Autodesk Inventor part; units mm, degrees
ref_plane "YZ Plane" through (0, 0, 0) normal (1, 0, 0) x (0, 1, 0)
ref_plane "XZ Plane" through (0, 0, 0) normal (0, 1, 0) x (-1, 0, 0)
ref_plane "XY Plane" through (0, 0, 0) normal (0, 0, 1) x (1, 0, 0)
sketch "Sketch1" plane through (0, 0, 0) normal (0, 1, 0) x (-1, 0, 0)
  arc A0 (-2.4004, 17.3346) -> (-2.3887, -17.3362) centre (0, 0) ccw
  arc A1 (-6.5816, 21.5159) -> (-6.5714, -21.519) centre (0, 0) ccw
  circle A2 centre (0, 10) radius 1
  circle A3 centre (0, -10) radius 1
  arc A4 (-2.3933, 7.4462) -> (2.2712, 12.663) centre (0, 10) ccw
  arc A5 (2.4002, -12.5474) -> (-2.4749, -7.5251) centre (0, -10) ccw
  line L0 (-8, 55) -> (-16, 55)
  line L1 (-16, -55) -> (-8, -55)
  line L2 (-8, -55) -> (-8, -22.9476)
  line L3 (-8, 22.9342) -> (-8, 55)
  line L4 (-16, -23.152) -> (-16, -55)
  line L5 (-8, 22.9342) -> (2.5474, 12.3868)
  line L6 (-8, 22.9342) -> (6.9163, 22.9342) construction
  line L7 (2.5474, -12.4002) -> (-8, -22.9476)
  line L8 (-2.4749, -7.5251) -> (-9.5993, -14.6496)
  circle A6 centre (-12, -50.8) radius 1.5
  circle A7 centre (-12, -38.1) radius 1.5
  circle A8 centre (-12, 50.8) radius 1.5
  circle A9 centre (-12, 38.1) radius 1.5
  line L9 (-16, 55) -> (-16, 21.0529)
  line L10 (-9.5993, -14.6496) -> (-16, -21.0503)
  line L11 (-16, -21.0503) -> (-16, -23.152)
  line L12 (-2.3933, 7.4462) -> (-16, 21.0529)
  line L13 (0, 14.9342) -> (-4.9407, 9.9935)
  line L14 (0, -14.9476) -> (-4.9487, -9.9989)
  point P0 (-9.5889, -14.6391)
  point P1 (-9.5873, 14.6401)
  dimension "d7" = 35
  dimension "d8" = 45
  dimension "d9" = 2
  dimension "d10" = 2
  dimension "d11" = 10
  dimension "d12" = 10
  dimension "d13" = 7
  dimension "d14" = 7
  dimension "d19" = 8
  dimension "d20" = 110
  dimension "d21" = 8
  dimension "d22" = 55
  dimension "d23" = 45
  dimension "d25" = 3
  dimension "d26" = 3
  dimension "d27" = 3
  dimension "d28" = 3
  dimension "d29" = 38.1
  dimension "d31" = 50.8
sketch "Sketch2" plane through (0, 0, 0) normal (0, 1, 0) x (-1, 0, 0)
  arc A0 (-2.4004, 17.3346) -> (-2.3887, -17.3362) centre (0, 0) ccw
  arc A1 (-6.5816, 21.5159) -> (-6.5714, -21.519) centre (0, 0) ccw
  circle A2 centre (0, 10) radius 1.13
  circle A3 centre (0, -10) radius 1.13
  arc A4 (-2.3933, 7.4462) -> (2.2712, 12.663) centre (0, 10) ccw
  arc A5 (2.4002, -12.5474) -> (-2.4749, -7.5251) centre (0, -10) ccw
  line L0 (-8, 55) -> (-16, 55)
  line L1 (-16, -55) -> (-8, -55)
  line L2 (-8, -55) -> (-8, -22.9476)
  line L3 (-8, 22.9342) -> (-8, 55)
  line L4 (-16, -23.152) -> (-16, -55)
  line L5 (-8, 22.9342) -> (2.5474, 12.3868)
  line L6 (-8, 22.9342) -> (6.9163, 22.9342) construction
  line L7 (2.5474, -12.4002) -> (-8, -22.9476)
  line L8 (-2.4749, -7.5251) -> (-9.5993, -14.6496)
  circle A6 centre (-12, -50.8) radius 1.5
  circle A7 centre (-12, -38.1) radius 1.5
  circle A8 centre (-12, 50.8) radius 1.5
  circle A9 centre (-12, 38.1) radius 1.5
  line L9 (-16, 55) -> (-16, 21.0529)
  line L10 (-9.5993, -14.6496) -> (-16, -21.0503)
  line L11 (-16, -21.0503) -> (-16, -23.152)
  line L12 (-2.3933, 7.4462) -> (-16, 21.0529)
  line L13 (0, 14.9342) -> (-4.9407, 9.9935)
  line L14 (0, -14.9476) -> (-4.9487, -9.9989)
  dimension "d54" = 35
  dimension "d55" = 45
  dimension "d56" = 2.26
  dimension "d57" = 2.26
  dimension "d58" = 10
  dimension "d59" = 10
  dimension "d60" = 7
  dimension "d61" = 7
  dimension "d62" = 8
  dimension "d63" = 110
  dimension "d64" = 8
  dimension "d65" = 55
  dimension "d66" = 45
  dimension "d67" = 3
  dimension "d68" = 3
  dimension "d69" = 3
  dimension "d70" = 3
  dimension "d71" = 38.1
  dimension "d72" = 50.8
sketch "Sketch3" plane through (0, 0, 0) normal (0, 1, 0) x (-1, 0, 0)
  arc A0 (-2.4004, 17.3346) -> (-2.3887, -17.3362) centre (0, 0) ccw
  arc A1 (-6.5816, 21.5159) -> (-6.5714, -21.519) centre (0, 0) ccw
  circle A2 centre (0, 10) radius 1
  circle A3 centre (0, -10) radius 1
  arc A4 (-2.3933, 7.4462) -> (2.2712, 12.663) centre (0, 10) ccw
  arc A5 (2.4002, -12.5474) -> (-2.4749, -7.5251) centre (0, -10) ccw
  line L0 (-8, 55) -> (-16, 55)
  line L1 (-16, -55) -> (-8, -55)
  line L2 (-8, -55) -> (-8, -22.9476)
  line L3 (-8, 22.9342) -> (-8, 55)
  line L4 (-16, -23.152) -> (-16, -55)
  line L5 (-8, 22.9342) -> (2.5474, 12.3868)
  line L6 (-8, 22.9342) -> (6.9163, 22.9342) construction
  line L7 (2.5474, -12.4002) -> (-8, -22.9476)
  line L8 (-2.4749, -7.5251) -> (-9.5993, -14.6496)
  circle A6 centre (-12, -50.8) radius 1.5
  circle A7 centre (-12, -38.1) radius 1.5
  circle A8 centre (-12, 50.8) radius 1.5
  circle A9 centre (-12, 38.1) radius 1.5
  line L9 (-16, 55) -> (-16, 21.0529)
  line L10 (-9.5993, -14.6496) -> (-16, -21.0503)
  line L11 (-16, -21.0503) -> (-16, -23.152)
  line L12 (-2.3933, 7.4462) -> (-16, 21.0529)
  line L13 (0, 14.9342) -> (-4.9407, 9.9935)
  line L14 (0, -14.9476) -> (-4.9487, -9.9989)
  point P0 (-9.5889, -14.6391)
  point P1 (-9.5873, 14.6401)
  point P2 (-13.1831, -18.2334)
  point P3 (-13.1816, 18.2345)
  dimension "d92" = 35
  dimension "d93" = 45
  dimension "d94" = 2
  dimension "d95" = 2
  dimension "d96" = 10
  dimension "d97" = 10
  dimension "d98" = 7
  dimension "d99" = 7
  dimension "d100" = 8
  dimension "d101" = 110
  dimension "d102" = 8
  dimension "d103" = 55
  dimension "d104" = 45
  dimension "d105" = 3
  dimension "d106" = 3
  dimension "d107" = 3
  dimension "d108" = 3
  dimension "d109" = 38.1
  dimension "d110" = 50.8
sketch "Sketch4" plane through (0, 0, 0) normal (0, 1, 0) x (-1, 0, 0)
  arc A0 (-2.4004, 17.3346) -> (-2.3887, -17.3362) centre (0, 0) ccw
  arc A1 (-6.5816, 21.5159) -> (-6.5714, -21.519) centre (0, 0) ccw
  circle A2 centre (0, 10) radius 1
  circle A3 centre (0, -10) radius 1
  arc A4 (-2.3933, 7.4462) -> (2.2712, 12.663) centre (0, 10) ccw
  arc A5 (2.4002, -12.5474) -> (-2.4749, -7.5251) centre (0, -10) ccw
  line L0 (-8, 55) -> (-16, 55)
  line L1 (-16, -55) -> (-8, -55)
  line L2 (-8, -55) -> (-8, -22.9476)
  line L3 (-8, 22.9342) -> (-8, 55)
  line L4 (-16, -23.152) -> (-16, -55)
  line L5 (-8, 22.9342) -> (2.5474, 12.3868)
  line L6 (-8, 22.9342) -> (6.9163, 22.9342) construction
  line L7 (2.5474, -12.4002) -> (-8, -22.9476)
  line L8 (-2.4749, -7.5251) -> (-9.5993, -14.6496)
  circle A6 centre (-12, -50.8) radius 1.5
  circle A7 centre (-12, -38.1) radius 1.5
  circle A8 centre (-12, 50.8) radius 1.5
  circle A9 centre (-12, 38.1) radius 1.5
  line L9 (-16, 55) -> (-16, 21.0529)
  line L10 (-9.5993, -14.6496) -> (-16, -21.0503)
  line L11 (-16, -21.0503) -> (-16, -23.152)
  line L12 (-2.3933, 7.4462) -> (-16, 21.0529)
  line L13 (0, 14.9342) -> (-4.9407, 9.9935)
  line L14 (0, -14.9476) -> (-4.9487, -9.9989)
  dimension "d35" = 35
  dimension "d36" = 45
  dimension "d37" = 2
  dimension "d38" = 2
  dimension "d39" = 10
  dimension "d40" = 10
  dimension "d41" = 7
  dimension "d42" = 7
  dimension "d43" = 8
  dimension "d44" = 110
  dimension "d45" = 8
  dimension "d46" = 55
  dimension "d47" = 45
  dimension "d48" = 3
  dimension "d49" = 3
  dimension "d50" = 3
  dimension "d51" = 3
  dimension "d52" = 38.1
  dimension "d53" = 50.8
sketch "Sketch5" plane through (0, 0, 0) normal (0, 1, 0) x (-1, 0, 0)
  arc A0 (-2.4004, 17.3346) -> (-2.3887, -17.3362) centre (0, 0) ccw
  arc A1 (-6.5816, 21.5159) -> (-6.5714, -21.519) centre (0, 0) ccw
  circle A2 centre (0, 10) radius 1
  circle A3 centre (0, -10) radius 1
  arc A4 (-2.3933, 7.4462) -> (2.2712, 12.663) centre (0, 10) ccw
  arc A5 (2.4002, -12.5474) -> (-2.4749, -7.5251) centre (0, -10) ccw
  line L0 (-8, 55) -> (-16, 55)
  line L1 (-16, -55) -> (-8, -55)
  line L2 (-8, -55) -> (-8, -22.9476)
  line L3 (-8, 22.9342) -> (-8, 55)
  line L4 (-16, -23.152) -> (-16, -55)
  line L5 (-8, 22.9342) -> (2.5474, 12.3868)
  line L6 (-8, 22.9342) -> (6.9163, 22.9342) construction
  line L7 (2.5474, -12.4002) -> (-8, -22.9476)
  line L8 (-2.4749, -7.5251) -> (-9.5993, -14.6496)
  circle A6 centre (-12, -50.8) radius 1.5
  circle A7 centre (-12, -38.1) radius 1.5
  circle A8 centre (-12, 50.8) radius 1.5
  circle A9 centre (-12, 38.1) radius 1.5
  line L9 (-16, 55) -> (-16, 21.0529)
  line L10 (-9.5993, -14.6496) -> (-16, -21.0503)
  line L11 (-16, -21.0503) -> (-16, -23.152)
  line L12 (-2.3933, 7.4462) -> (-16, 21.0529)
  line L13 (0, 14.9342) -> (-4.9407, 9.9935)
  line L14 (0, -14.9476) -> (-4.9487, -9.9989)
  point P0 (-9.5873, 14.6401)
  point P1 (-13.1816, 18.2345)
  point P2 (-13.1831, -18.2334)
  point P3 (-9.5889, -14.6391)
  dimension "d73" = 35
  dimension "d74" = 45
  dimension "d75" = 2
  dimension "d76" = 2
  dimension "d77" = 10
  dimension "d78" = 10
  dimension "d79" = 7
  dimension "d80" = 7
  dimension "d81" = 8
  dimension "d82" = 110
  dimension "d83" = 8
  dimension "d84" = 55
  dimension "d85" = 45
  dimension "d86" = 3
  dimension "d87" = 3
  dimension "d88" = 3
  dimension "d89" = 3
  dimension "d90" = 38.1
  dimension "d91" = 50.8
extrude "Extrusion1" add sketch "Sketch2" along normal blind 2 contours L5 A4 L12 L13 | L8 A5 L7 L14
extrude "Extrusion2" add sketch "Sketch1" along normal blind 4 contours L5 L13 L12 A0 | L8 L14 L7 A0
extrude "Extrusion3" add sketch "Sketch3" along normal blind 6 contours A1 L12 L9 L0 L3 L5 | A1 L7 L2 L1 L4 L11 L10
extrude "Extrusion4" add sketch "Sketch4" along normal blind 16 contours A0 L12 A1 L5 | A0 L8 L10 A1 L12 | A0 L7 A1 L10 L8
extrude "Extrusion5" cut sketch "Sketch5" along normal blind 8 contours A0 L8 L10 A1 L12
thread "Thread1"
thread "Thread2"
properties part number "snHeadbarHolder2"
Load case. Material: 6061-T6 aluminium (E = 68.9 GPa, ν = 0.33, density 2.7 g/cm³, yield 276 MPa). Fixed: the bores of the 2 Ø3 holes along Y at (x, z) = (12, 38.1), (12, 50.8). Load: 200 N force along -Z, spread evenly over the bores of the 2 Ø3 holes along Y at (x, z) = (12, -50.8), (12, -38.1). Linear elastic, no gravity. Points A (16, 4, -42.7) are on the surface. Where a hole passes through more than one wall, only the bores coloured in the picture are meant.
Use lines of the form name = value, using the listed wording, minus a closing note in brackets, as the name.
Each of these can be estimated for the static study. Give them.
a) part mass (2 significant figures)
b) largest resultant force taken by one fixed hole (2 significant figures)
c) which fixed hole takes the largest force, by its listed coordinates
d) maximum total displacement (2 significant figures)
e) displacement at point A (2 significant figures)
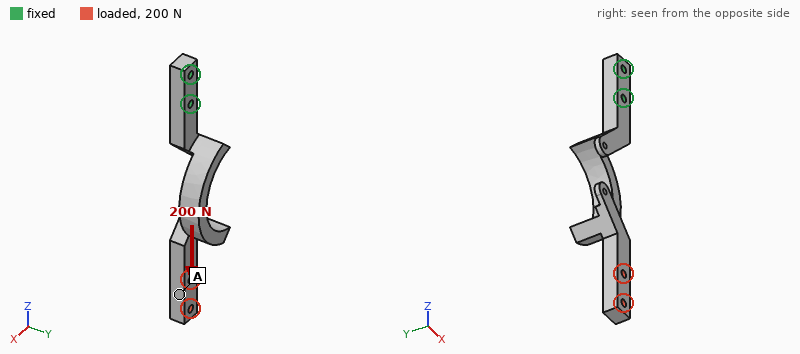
part mass = 17 g
largest resultant force taken by one fixed hole = 190 N
which fixed hole takes the largest force, by its listed coordinates = (12, 38.1)
maximum total displacement = 0.63 mm
displacement at point A = 0.48 mm
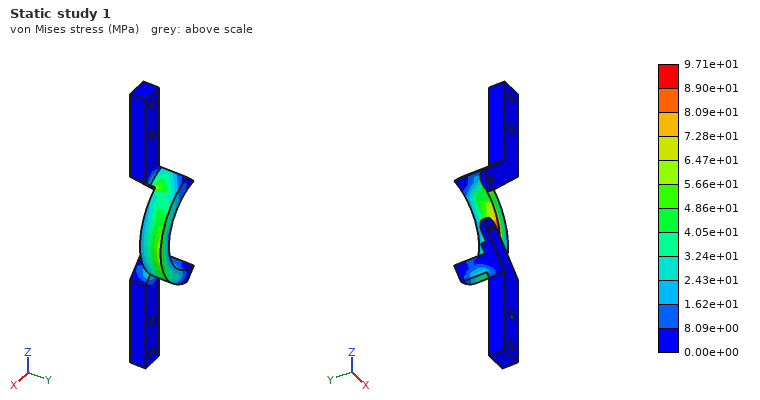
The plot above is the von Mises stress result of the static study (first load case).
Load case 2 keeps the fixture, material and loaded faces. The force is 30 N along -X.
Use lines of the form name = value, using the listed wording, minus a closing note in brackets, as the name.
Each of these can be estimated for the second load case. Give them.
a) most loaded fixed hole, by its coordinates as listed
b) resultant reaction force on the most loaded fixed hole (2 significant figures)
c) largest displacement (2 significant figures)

most loaded fixed hole, by its coordinates as listed = (12, 38.1)
resultant reaction force on the most loaded fixed hole = 110 N
largest displacement = 1.0 mm
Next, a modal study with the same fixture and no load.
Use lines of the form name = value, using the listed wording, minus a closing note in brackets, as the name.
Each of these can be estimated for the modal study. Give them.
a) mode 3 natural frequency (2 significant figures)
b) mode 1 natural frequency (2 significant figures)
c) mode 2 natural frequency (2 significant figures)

mode 3 natural frequency = 2000 Hz
mode 1 natural frequency = 450 Hz
mode 2 natural frequency = 460 Hz
